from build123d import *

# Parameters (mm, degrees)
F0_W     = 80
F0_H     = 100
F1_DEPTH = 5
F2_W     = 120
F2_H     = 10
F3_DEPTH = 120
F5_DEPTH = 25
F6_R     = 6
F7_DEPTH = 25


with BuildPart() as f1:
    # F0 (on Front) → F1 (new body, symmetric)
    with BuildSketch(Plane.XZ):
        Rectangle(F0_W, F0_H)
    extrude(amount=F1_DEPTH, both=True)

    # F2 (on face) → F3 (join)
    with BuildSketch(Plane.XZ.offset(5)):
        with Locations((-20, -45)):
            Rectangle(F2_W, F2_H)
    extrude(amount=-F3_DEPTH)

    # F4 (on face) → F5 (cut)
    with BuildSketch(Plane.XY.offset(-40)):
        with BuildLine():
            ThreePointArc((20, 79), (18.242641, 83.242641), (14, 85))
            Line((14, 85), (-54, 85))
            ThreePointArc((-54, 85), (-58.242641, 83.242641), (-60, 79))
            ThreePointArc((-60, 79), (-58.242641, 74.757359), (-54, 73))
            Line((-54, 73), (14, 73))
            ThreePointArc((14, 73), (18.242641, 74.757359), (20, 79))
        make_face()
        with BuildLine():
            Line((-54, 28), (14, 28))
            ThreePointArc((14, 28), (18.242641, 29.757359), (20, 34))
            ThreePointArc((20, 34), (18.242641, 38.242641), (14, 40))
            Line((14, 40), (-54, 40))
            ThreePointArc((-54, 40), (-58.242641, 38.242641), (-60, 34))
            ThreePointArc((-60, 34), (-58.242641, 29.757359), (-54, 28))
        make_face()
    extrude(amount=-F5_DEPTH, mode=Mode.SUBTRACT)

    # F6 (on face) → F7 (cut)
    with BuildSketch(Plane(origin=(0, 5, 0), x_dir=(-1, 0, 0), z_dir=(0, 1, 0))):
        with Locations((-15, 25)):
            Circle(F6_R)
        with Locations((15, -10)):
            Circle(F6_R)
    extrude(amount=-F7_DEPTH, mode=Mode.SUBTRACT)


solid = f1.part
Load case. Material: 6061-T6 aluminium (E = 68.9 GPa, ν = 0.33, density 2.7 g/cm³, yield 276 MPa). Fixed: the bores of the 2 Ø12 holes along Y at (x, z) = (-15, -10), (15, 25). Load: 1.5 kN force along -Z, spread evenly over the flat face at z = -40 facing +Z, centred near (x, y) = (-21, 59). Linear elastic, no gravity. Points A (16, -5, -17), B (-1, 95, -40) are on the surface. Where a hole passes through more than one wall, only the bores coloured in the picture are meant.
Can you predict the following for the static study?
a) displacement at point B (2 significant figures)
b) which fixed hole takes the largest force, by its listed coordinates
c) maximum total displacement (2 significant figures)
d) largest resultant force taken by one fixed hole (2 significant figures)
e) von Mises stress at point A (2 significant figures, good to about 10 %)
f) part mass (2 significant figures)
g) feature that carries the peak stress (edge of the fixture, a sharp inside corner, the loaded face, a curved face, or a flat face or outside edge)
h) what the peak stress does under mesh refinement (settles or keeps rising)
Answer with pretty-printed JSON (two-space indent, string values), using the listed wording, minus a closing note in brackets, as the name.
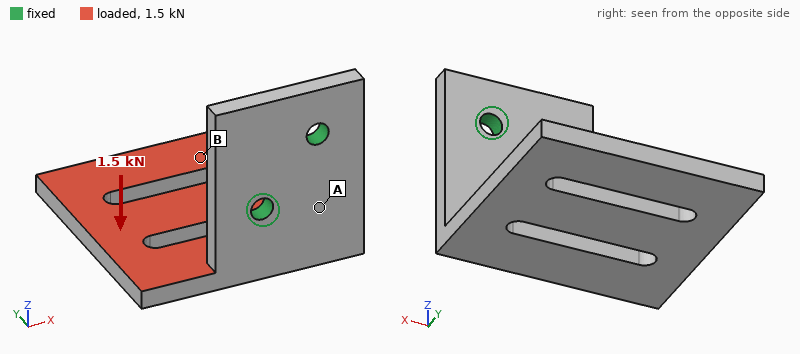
{
  "displacement at point B": "1.3 mm",
  "which fixed hole takes the largest force, by its listed coordinates": "(-15, -10)",
  "maximum total displacement": "1.8 mm",
  "largest resultant force taken by one fixed hole": "1.7 kN",
  "von Mises stress at point A": "42 MPa",
  "part mass": "530 g",
  "feature that carries the peak stress": "edge of the fixture",
  "what the peak stress does under mesh refinement": "keeps rising"
}
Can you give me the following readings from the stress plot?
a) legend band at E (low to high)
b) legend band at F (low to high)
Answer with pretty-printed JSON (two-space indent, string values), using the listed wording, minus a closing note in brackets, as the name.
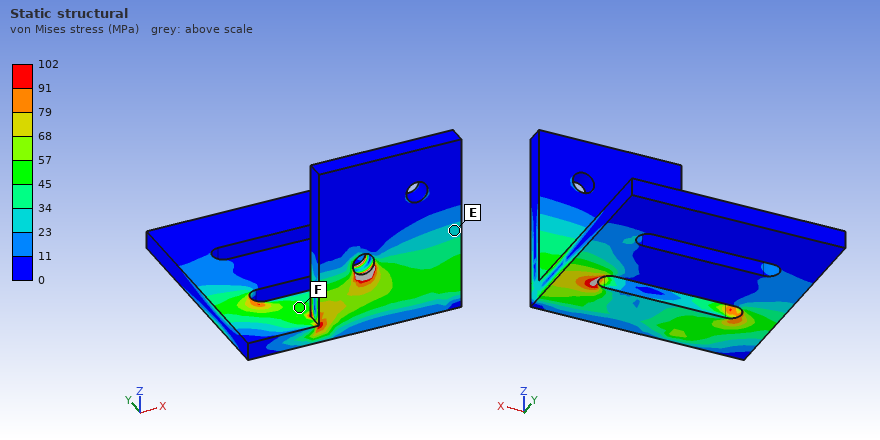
{
  "legend band at E": "23 to 34 MPa",
  "legend band at F": "45 to 57 MPa"
}
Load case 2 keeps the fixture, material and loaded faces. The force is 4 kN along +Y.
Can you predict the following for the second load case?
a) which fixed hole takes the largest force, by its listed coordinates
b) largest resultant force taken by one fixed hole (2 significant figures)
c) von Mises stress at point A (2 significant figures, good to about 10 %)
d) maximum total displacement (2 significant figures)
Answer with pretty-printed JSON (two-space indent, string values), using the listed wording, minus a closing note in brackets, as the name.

{
  "which fixed hole takes the largest force, by its listed coordinates": "(-15, -10)",
  "largest resultant force taken by one fixed hole": "4.7 kN",
  "von Mises stress at point A": "29 MPa",
  "maximum total displacement": "0.37 mm"
}
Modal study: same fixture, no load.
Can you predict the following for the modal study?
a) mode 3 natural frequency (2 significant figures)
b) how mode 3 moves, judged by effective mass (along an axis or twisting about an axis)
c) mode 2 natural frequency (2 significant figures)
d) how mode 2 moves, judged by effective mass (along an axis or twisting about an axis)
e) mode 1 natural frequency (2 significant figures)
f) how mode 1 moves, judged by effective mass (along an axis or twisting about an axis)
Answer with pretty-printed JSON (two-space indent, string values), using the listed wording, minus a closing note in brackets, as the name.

{
  "mode 3 natural frequency": "1000 Hz",
  "how mode 3 moves, judged by effective mass": "twisting about Y",
  "mode 2 natural frequency": "550 Hz",
  "how mode 2 moves, judged by effective mass": "along X",
  "mode 1 natural frequency": "320 Hz",
  "how mode 1 moves, judged by effective mass": "along Z"
}
